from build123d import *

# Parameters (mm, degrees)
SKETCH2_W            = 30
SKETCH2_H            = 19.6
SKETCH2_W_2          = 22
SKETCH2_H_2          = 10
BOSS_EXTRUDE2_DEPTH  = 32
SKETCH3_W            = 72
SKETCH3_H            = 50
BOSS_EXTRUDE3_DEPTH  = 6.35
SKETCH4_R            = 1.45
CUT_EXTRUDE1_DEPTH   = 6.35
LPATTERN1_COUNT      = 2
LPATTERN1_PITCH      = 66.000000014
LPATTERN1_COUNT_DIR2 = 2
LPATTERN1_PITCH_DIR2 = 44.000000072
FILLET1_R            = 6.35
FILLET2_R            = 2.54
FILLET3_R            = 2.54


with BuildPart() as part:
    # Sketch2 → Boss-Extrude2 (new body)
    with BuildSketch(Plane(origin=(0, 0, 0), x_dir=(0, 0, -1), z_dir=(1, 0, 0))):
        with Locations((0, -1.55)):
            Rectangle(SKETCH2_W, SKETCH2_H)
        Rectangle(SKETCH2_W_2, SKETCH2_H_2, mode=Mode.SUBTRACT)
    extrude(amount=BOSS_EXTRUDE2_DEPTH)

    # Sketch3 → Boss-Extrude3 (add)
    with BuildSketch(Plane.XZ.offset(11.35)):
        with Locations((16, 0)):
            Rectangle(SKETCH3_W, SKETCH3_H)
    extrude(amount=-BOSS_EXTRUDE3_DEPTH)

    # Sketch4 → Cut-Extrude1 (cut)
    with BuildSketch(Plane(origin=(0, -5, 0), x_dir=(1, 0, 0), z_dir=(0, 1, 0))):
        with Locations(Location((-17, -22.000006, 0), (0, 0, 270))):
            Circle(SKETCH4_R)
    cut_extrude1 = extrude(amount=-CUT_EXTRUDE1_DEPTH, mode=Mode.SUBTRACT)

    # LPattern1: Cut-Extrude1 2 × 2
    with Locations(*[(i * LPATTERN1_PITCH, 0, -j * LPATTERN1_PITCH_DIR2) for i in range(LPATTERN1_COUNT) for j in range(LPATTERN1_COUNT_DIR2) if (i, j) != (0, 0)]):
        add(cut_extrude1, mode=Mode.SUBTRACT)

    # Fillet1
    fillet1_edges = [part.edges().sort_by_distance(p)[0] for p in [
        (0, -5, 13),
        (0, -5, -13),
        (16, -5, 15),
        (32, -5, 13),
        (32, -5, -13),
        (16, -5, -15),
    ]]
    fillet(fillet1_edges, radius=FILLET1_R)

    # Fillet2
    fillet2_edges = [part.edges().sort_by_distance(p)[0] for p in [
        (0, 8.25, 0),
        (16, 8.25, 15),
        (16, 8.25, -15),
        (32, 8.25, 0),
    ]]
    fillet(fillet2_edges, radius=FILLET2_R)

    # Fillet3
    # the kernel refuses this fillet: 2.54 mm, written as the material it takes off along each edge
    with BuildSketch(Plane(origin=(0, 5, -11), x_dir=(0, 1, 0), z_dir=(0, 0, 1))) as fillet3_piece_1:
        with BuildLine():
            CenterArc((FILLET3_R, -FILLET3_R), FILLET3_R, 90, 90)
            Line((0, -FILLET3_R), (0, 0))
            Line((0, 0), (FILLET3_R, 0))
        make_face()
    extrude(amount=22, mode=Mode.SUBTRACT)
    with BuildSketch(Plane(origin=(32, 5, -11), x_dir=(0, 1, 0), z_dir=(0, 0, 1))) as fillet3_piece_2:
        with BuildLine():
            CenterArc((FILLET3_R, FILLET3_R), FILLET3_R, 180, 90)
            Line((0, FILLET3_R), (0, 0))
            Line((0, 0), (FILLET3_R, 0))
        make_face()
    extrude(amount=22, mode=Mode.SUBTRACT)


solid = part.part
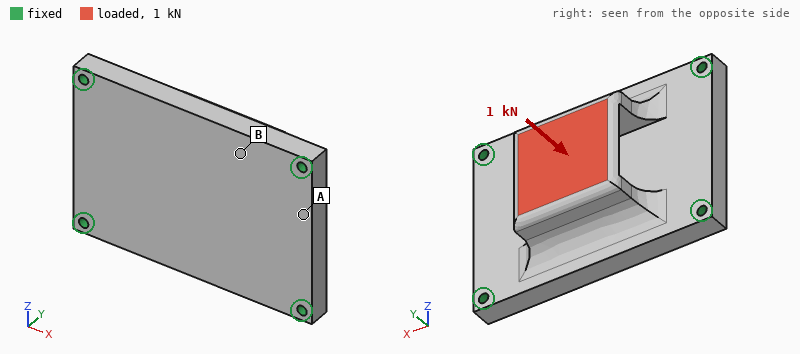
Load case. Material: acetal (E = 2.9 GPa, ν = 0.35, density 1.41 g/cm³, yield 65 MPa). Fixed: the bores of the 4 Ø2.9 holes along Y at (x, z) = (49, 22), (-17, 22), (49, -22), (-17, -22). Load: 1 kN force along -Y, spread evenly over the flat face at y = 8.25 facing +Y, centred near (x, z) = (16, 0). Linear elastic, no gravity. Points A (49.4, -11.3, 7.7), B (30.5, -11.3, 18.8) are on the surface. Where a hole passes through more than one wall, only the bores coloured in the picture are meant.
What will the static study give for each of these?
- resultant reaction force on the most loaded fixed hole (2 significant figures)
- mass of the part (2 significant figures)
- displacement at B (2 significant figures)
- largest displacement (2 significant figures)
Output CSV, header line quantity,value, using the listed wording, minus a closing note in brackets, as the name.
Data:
quantity,value
resultant reaction force on the most loaded fixed hole,270 N
mass of the part,41 g
displacement at B,0.27 mm
largest displacement,0.54 mm
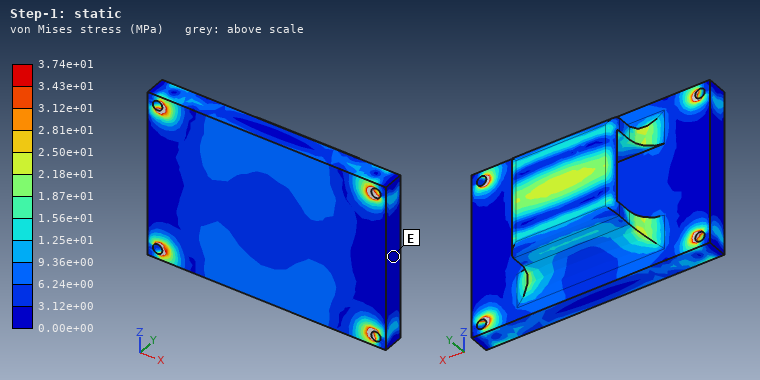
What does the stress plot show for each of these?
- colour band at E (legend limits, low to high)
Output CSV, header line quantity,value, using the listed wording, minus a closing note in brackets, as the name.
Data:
quantity,value
colour band at E,0.00e+00 to 3.12e+00 MPa
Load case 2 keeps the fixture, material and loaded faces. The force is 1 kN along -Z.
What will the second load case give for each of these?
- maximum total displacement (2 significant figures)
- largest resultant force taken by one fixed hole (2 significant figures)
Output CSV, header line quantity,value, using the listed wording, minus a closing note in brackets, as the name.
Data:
quantity,value
maximum total displacement,0.50 mm
largest resultant force taken by one fixed hole,390 N
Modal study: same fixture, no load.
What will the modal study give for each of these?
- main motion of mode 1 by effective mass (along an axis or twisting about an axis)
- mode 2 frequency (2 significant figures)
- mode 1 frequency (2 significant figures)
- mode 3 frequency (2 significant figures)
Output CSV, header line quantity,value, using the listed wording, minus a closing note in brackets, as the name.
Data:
quantity,value
main motion of mode 1 by effective mass,along Y
mode 2 frequency,2300 Hz
mode 1 frequency,1700 Hz
mode 3 frequency,3400 Hz
